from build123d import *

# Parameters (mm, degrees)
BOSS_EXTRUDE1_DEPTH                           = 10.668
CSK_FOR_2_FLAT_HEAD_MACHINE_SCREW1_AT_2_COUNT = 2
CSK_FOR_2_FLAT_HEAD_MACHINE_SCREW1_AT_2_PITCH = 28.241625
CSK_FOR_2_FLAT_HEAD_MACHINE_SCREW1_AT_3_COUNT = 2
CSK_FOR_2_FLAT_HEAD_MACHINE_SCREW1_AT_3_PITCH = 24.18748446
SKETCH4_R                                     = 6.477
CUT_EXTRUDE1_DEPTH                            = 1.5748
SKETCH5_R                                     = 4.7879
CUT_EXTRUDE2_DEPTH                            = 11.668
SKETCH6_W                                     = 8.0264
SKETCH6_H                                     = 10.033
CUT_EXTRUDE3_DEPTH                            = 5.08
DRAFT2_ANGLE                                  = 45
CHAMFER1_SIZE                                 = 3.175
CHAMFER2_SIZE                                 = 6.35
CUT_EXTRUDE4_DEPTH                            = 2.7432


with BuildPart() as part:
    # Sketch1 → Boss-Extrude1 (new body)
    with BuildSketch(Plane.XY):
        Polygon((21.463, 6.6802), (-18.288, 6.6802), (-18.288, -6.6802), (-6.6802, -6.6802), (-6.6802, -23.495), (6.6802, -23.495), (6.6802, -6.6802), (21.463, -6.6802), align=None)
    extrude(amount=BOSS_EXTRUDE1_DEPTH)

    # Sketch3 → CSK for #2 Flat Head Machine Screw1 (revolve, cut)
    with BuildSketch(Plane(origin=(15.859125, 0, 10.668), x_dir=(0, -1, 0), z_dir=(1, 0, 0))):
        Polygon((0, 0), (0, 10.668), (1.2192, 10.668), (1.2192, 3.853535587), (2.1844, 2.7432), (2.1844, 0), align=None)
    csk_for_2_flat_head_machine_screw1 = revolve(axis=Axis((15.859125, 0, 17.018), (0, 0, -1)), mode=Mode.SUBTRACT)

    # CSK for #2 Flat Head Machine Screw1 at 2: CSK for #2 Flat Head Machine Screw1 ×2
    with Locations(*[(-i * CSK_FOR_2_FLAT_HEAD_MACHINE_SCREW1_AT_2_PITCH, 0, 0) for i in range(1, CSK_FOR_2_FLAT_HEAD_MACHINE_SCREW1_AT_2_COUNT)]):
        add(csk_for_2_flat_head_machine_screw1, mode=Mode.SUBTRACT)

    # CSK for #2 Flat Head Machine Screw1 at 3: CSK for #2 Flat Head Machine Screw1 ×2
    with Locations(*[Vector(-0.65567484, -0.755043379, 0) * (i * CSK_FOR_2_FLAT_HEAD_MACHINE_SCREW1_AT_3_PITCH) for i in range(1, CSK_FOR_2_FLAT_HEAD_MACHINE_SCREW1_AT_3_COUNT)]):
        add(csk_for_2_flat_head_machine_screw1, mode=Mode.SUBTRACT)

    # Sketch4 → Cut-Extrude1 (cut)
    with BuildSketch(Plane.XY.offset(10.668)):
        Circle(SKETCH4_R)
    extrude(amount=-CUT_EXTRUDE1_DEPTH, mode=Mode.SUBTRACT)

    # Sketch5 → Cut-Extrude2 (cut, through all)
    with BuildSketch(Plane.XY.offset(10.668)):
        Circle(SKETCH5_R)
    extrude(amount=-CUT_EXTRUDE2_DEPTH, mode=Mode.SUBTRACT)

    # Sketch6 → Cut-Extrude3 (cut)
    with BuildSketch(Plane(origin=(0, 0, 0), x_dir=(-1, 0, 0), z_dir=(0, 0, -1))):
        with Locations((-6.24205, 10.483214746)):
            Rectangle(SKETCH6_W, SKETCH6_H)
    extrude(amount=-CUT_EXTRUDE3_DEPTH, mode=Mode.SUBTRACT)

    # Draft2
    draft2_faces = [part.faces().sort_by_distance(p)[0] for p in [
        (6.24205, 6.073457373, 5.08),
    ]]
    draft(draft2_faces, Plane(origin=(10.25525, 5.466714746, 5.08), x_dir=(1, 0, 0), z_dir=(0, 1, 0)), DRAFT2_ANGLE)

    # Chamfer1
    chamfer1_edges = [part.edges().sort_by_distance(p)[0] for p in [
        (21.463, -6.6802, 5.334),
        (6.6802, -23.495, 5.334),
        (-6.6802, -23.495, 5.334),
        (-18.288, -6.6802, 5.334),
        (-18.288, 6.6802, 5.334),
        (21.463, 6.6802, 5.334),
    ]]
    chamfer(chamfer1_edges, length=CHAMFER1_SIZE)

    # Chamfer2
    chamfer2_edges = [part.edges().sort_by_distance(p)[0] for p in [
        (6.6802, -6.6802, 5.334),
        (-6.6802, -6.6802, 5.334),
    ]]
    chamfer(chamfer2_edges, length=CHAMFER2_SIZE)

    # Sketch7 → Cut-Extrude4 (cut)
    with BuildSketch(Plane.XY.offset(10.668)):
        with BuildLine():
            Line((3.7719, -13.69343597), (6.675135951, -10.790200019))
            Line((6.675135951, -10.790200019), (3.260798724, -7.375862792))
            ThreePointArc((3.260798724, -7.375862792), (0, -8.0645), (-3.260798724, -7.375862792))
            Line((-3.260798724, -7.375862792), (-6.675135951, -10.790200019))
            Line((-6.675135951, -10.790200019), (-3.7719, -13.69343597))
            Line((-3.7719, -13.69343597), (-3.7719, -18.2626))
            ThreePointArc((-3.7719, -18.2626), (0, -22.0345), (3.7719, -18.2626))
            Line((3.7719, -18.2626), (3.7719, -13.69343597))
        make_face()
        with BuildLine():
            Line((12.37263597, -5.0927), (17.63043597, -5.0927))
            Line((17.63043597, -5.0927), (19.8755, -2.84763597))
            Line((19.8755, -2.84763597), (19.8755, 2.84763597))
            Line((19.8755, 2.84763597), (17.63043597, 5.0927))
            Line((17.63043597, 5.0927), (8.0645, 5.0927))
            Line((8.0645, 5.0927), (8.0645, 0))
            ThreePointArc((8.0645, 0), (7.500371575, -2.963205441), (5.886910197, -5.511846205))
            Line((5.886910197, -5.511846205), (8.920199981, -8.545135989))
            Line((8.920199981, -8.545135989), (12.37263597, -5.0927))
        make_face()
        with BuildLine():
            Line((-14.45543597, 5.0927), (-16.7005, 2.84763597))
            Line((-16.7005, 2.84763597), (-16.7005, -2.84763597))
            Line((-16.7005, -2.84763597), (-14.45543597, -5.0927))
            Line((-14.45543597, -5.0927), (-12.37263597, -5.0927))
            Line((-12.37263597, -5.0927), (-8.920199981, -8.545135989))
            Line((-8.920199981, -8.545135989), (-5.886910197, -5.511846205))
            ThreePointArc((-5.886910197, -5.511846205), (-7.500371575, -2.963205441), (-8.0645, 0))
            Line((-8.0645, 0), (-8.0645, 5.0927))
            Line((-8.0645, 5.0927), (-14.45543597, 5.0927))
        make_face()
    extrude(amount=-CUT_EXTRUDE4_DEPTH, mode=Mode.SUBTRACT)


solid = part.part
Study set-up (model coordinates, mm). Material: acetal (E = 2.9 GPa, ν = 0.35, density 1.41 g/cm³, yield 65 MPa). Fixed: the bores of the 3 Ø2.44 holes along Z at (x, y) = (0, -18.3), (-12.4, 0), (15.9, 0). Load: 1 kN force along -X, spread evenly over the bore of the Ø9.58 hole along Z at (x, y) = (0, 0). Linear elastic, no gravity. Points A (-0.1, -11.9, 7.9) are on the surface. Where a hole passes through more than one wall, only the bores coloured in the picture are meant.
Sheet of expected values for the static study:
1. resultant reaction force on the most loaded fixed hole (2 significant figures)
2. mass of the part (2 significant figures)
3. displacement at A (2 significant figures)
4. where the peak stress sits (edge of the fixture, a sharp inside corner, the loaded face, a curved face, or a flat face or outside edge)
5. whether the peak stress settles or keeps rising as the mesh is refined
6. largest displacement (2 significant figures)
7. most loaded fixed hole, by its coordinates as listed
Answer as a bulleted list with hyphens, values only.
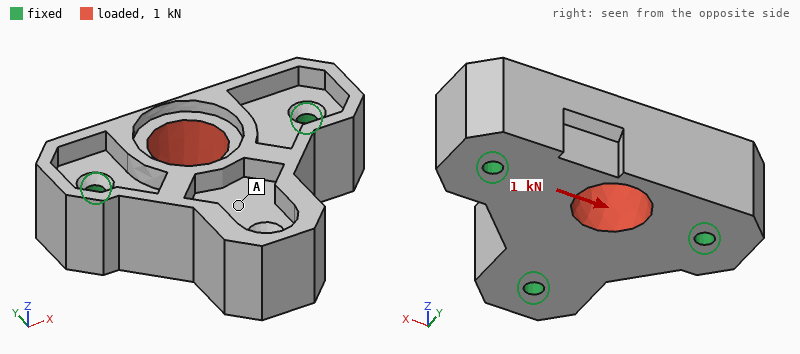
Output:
- 500 N
- 8.7 g
- 11 µm
- edge of the fixture
- keeps rising
- 32 µm
- (-12.4, 0)
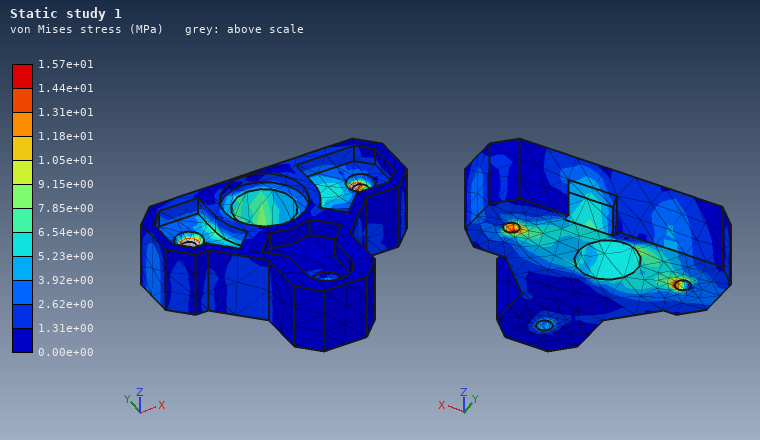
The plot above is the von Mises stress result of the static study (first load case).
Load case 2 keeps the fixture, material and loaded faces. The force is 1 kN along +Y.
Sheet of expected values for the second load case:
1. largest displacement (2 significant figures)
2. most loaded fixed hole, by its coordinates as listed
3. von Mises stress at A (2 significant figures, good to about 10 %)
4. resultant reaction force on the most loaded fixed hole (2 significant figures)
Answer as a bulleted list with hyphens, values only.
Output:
- 94 µm
- (0, -18.3)
- 7.7 MPa
- 490 N
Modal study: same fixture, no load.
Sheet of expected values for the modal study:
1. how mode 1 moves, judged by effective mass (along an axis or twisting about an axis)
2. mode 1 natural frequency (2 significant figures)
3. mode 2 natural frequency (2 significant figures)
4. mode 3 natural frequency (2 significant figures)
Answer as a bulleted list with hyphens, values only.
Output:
- along Z
- 9200 Hz
- 12 kHz
- 12 kHz
